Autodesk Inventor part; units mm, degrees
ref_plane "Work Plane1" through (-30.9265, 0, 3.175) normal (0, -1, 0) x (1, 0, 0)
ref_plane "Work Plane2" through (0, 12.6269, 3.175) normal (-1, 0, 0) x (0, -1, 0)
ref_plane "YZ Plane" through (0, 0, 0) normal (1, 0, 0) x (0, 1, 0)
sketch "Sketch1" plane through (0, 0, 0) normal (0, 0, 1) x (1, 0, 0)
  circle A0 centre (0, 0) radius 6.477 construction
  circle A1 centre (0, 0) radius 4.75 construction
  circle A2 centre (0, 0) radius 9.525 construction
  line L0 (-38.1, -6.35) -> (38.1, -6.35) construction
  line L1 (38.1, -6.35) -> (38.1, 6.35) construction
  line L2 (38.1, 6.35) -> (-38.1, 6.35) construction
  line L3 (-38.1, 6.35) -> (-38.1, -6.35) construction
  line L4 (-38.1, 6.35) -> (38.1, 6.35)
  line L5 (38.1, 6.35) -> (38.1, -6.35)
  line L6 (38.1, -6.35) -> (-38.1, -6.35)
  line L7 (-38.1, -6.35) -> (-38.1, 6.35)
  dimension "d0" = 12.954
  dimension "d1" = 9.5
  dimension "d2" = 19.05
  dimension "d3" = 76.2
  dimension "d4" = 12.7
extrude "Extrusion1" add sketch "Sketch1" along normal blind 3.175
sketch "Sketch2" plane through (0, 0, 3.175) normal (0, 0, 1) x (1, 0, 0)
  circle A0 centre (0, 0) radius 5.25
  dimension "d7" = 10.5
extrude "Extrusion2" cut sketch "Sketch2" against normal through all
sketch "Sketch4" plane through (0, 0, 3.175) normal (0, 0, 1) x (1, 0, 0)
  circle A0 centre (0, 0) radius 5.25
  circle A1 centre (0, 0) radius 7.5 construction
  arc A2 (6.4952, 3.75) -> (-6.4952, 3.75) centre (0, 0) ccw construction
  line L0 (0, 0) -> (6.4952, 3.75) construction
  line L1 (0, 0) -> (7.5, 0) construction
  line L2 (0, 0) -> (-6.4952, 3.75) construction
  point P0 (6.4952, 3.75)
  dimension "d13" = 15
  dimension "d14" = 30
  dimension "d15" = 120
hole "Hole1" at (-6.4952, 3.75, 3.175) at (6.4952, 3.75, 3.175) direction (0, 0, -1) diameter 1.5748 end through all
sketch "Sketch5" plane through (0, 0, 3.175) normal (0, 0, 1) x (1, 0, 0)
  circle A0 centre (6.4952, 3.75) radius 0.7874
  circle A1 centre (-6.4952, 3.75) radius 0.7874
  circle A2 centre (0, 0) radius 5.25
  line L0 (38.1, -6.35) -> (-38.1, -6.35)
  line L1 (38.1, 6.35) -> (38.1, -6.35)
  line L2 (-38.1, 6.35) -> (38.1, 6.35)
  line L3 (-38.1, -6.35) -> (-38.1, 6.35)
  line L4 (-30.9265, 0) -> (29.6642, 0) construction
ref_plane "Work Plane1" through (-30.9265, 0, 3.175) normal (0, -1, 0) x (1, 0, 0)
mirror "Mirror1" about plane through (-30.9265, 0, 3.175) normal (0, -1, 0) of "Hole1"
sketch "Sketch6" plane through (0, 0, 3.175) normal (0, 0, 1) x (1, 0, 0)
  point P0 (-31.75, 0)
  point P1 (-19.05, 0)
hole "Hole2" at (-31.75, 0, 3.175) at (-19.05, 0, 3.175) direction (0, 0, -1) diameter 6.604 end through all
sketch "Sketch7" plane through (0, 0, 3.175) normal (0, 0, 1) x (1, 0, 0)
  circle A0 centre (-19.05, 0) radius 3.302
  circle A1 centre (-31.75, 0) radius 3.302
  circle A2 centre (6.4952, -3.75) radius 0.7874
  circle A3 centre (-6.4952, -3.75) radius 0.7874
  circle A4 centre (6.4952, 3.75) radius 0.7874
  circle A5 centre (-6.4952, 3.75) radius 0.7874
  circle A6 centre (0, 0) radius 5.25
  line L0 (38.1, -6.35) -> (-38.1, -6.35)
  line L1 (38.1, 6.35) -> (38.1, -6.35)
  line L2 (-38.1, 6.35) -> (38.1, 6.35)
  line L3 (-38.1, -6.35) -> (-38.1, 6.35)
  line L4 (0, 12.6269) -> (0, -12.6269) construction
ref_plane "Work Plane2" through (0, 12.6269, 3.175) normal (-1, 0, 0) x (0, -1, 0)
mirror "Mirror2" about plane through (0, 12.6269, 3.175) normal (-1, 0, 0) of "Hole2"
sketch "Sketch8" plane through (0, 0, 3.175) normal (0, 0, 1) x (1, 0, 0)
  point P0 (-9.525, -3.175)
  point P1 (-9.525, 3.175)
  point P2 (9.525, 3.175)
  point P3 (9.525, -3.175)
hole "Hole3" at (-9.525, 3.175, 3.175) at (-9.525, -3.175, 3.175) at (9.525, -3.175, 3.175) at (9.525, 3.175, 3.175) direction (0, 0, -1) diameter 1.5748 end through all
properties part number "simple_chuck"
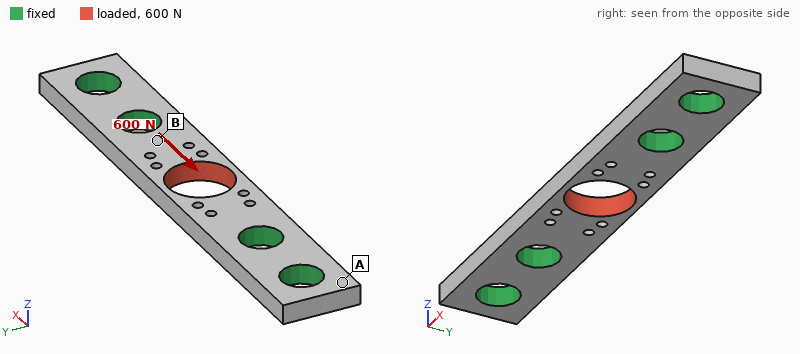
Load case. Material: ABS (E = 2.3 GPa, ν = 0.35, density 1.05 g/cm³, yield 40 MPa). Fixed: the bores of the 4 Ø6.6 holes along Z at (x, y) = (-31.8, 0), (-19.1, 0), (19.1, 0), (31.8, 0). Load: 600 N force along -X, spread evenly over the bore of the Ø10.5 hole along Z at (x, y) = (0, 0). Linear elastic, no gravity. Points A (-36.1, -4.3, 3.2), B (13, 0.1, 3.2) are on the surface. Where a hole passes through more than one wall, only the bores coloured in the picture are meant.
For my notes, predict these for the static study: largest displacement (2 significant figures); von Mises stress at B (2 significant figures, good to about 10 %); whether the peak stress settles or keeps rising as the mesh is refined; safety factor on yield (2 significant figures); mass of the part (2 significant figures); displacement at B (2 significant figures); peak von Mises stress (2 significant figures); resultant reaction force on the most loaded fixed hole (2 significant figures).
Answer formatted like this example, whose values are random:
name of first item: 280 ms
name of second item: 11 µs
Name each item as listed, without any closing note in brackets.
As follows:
largest displacement: 72 µm
von Mises stress at B: 9.8 MPa
whether the peak stress settles or keeps rising as the mesh is refined: settles
safety factor on yield: 1.5
mass of the part: 2.4 g
displacement at B: 12 µm
peak von Mises stress: 26 MPa
resultant reaction force on the most loaded fixed hole: 290 N
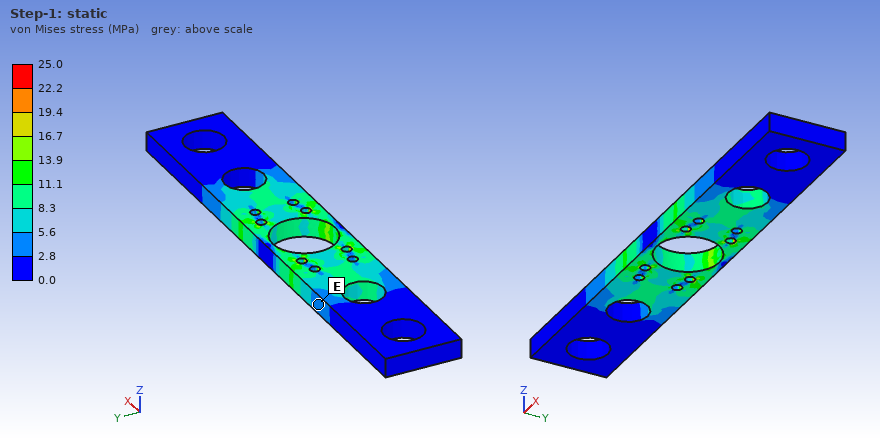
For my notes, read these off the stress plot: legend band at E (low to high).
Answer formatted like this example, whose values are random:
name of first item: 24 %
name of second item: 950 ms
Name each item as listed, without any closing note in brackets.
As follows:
legend band at E: 2.8 to 5.6 MPa
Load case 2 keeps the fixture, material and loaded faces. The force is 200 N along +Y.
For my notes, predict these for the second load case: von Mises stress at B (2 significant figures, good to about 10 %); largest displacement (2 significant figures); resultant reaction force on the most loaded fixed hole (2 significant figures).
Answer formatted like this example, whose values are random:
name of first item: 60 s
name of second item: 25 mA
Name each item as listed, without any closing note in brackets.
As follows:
von Mises stress at B: 6.1 MPa
largest displacement: 0.13 mm
resultant reaction force on the most loaded fixed hole: 110 N
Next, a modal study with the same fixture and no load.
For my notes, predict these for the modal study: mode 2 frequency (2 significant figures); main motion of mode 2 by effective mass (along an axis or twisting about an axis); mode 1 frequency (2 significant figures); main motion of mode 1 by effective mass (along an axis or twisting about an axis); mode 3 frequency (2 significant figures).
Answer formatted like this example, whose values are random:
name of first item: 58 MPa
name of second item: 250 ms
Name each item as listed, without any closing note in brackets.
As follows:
mode 2 frequency: 7000 Hz
main motion of mode 2 by effective mass: twisting about X
mode 1 frequency: 4800 Hz
main motion of mode 1 by effective mass: along Z
mode 3 frequency: 9300 Hz
